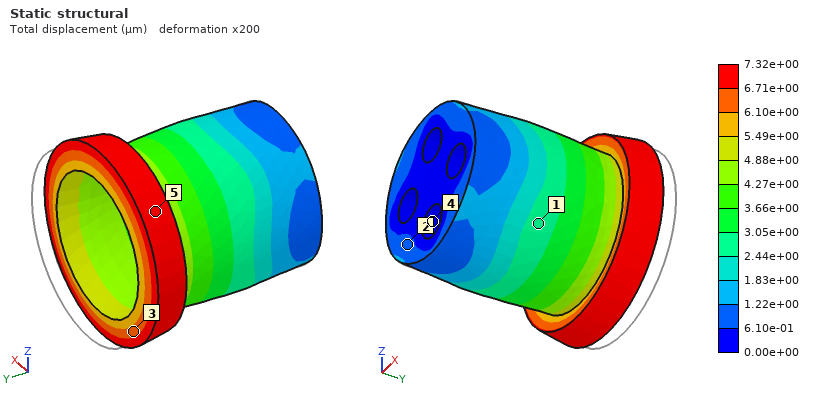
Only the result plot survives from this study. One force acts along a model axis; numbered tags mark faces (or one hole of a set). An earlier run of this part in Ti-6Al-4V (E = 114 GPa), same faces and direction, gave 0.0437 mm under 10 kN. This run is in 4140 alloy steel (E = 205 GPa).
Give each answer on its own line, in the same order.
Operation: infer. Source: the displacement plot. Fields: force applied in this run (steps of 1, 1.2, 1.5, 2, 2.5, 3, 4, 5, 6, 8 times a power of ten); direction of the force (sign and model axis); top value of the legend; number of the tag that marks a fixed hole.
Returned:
3 kN
-Y
7.32e+00 µm
4
